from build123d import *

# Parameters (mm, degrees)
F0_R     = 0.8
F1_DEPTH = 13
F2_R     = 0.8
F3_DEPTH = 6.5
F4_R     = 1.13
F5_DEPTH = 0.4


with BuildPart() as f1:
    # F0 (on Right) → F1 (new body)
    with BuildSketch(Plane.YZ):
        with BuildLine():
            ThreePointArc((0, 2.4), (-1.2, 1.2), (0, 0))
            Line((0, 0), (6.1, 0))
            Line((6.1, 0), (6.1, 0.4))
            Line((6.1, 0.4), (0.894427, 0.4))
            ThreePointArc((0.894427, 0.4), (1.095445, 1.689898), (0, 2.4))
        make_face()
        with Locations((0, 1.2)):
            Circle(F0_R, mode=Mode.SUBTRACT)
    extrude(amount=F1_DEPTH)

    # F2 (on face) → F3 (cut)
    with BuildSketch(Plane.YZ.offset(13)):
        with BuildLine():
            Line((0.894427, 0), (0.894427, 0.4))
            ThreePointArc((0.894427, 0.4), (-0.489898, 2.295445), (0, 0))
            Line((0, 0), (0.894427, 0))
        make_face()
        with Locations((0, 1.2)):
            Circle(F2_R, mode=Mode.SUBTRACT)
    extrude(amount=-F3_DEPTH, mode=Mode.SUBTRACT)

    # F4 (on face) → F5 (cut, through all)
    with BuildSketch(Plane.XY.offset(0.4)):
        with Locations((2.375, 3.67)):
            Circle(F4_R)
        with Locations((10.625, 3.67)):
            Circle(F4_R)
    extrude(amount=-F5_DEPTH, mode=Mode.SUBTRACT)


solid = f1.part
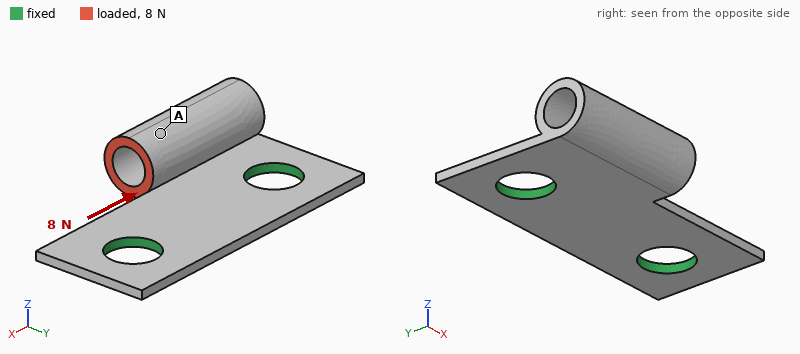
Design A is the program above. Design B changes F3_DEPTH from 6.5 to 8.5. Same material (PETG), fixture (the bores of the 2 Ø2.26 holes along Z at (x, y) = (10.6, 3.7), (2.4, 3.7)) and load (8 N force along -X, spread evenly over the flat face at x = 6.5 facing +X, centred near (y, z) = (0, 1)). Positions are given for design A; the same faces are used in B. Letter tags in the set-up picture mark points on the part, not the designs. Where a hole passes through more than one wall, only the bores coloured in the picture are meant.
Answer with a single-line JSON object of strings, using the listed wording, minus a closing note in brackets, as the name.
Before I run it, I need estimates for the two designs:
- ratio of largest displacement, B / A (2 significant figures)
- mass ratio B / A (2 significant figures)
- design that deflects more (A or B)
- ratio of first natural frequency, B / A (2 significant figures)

{"ratio of largest displacement, B / A": "1.5", "mass ratio B / A": "0.87", "design that deflects more": "B", "ratio of first natural frequency, B / A": "1.1"}
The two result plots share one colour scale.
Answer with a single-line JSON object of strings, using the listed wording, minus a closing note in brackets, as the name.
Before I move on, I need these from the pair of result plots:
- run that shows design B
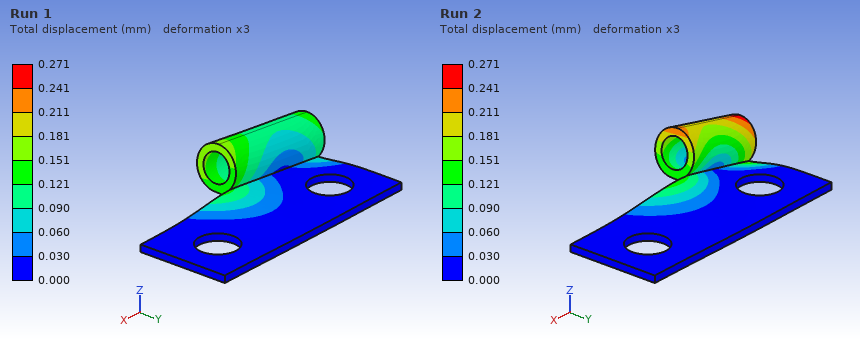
{"run that shows design B": "Run 2"}
